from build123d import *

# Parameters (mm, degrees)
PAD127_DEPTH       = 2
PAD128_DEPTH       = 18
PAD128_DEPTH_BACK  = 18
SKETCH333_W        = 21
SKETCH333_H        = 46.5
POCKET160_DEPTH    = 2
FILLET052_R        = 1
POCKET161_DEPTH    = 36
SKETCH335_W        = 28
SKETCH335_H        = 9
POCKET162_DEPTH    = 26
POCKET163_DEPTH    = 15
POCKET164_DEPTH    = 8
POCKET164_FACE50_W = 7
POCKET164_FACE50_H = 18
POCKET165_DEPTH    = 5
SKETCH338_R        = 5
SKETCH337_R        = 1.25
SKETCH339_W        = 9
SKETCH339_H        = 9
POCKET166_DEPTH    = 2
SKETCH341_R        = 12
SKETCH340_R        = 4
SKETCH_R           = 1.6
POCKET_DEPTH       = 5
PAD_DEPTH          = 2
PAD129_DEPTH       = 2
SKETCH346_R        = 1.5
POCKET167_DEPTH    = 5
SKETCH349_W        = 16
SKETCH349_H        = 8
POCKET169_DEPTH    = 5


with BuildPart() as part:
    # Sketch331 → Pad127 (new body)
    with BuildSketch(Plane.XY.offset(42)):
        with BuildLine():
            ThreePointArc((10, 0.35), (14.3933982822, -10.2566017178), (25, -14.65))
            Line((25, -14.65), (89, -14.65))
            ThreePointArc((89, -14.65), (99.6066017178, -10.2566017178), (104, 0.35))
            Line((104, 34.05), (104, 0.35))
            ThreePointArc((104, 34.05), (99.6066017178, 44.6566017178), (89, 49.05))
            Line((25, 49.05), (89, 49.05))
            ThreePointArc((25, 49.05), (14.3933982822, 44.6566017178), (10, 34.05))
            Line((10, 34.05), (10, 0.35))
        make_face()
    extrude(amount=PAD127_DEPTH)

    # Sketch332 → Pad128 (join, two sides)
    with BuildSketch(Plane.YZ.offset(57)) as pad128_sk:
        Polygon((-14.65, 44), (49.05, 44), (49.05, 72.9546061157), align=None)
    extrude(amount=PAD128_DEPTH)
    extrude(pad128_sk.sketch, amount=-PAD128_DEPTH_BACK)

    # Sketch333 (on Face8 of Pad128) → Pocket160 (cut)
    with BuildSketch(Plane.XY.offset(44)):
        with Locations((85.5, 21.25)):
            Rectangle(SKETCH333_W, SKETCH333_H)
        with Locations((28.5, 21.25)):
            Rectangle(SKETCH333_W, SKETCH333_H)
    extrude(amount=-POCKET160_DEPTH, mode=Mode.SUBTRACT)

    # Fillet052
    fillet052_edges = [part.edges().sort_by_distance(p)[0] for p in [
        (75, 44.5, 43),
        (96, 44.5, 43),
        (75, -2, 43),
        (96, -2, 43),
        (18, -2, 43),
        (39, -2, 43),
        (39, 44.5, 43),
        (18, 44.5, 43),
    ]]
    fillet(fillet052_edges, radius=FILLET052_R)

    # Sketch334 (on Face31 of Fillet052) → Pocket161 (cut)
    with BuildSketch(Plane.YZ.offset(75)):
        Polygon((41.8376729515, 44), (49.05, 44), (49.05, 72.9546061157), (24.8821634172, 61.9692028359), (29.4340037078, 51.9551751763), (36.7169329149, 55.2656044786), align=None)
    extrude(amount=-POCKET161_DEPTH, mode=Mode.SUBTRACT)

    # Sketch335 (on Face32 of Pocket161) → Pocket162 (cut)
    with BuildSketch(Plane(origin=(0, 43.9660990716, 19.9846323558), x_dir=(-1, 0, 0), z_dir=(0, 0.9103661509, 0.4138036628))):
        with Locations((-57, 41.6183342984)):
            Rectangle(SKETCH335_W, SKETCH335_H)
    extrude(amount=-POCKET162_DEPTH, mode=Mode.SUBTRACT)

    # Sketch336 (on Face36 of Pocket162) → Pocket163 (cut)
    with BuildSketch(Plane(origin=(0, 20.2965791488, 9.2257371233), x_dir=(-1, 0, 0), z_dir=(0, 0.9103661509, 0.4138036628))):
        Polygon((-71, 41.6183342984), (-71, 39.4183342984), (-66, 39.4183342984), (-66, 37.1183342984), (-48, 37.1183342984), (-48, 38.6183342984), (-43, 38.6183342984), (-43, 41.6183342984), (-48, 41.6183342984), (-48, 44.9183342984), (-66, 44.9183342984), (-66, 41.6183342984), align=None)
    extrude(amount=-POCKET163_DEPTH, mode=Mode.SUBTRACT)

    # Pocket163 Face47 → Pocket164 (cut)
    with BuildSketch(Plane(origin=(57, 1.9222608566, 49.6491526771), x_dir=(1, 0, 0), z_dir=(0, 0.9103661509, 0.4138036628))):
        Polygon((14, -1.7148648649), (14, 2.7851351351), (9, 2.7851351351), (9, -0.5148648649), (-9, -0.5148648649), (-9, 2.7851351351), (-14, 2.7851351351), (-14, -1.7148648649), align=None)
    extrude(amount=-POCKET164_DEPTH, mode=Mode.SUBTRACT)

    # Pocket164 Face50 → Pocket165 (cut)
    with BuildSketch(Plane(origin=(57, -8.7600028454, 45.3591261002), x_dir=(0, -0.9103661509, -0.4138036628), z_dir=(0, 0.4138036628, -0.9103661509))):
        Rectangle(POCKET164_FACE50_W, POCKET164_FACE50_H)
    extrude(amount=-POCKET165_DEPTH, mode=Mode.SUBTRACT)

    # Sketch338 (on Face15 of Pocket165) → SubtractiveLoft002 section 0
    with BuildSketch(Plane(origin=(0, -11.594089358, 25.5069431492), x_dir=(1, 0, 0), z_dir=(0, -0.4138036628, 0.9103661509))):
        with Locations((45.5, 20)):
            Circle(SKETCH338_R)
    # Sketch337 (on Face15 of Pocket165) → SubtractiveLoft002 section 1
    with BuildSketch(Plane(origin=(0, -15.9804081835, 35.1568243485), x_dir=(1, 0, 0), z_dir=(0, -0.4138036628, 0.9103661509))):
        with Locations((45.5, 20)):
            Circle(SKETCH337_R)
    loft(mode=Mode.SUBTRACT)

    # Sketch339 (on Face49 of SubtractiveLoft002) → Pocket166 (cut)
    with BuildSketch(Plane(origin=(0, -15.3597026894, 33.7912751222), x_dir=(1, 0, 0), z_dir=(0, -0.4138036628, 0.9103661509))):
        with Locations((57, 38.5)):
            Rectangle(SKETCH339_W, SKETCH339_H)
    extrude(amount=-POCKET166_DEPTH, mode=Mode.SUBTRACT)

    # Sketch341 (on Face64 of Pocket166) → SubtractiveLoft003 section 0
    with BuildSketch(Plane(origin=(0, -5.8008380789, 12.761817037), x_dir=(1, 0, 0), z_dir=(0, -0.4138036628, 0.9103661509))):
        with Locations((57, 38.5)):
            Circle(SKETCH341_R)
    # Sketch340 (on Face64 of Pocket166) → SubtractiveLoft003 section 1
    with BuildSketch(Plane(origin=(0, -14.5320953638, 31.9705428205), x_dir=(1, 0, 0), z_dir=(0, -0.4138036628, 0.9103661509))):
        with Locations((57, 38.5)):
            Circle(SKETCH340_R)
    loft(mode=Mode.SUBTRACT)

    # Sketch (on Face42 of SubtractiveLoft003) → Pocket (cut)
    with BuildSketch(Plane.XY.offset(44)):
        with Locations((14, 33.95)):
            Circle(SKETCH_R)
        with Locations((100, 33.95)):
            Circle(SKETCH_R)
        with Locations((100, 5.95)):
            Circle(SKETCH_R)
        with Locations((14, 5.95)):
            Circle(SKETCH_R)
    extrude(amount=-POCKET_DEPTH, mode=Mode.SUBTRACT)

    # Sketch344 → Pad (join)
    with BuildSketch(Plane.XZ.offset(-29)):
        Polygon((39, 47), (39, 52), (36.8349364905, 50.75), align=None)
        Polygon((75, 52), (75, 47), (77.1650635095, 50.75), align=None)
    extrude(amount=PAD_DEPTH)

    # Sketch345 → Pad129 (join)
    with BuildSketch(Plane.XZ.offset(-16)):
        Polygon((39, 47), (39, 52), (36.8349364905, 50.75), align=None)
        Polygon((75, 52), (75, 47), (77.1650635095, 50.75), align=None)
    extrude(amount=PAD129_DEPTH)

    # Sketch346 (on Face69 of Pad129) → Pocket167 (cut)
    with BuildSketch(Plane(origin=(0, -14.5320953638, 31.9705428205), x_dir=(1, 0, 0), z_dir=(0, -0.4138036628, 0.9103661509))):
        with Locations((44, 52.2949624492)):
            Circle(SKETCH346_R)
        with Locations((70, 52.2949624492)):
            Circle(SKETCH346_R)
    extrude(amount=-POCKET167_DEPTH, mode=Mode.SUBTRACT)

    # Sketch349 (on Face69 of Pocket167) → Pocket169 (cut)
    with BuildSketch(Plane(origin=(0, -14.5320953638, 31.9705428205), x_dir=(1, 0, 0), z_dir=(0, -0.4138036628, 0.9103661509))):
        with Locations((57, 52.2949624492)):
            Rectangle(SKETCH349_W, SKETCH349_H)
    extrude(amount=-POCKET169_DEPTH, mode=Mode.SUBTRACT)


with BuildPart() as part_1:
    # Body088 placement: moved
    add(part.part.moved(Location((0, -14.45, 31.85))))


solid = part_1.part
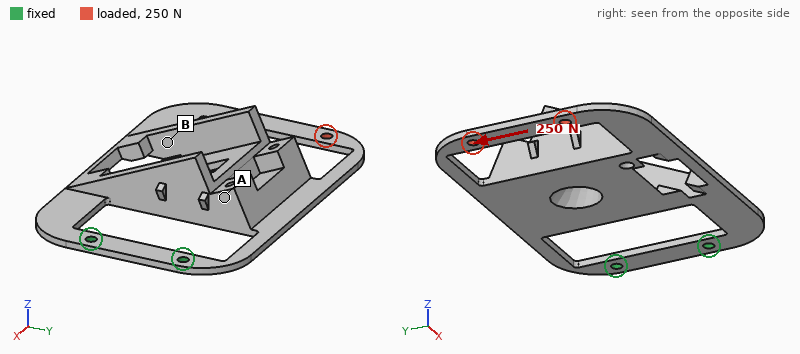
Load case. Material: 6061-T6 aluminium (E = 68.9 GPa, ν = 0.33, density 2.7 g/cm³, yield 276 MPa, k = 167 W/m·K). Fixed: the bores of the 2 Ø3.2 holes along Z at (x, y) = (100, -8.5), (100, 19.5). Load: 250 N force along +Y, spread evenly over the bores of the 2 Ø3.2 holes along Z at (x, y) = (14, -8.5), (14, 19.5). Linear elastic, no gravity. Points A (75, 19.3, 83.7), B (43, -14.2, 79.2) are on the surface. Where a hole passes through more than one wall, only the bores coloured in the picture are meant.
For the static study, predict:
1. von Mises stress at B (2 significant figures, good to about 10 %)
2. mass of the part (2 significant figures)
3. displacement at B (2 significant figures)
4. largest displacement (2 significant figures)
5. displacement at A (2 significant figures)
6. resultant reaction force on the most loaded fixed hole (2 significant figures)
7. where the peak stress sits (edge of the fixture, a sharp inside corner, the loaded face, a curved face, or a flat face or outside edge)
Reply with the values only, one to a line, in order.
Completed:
39 MPa
42 g
0.41 mm
0.70 mm
0.29 mm
520 N
a curved face
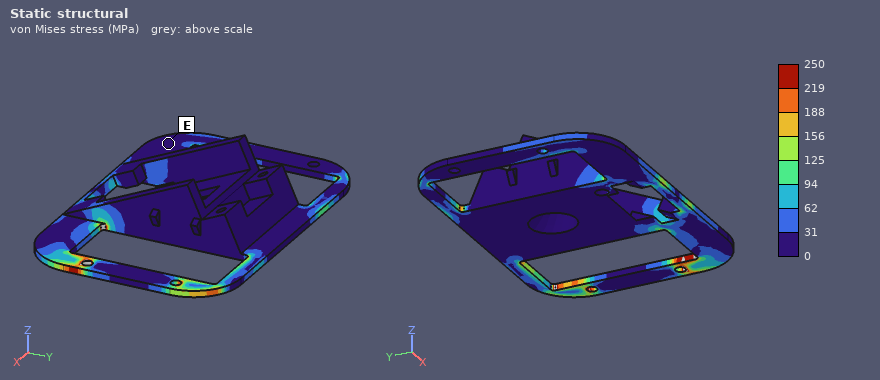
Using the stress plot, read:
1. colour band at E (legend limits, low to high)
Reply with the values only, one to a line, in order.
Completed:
0 to 31 MPa
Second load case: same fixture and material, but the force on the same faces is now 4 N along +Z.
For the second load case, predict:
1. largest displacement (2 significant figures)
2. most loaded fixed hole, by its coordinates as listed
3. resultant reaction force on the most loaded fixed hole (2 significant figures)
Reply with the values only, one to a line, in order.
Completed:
1.2 mm
(100, -8.5)
2.2 N
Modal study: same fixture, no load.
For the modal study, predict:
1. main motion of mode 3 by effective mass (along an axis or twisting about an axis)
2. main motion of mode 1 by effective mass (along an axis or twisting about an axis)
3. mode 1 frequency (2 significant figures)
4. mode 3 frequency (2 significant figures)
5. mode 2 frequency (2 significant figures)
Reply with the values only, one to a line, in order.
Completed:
along Y
along Z
91 Hz
790 Hz
510 Hz
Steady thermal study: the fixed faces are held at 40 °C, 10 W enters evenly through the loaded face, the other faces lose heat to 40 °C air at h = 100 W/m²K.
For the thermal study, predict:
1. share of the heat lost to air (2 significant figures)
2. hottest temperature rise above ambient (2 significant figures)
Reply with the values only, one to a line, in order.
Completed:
96 %
53 K
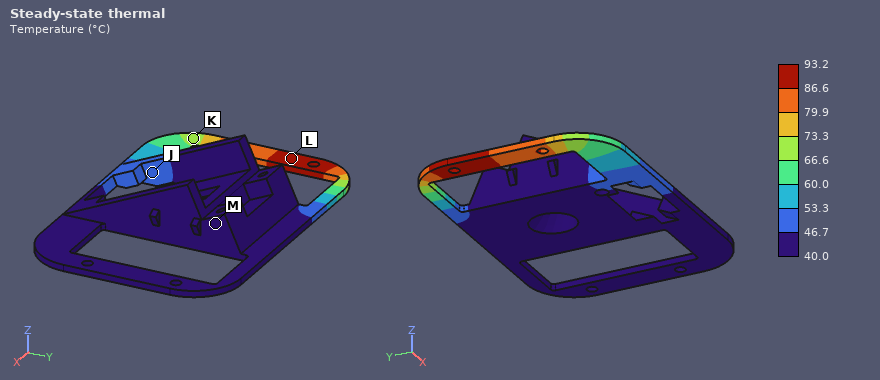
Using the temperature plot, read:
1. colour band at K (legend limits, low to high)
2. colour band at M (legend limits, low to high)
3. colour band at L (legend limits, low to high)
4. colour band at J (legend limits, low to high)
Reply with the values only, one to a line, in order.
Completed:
66.6 to 73.3 °C
40.0 to 46.7 °C
86.6 to 93.2 °C
46.7 to 53.3 °C
